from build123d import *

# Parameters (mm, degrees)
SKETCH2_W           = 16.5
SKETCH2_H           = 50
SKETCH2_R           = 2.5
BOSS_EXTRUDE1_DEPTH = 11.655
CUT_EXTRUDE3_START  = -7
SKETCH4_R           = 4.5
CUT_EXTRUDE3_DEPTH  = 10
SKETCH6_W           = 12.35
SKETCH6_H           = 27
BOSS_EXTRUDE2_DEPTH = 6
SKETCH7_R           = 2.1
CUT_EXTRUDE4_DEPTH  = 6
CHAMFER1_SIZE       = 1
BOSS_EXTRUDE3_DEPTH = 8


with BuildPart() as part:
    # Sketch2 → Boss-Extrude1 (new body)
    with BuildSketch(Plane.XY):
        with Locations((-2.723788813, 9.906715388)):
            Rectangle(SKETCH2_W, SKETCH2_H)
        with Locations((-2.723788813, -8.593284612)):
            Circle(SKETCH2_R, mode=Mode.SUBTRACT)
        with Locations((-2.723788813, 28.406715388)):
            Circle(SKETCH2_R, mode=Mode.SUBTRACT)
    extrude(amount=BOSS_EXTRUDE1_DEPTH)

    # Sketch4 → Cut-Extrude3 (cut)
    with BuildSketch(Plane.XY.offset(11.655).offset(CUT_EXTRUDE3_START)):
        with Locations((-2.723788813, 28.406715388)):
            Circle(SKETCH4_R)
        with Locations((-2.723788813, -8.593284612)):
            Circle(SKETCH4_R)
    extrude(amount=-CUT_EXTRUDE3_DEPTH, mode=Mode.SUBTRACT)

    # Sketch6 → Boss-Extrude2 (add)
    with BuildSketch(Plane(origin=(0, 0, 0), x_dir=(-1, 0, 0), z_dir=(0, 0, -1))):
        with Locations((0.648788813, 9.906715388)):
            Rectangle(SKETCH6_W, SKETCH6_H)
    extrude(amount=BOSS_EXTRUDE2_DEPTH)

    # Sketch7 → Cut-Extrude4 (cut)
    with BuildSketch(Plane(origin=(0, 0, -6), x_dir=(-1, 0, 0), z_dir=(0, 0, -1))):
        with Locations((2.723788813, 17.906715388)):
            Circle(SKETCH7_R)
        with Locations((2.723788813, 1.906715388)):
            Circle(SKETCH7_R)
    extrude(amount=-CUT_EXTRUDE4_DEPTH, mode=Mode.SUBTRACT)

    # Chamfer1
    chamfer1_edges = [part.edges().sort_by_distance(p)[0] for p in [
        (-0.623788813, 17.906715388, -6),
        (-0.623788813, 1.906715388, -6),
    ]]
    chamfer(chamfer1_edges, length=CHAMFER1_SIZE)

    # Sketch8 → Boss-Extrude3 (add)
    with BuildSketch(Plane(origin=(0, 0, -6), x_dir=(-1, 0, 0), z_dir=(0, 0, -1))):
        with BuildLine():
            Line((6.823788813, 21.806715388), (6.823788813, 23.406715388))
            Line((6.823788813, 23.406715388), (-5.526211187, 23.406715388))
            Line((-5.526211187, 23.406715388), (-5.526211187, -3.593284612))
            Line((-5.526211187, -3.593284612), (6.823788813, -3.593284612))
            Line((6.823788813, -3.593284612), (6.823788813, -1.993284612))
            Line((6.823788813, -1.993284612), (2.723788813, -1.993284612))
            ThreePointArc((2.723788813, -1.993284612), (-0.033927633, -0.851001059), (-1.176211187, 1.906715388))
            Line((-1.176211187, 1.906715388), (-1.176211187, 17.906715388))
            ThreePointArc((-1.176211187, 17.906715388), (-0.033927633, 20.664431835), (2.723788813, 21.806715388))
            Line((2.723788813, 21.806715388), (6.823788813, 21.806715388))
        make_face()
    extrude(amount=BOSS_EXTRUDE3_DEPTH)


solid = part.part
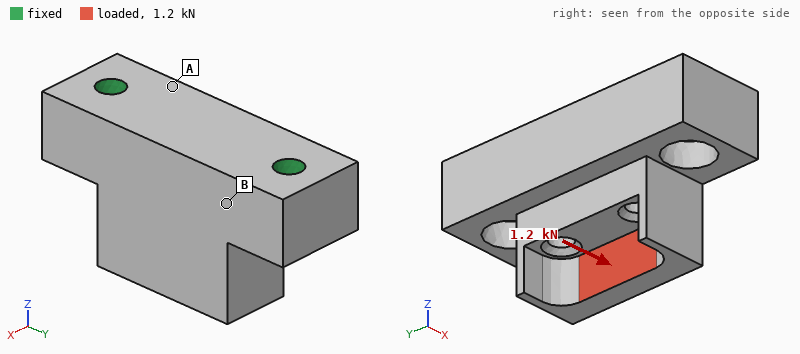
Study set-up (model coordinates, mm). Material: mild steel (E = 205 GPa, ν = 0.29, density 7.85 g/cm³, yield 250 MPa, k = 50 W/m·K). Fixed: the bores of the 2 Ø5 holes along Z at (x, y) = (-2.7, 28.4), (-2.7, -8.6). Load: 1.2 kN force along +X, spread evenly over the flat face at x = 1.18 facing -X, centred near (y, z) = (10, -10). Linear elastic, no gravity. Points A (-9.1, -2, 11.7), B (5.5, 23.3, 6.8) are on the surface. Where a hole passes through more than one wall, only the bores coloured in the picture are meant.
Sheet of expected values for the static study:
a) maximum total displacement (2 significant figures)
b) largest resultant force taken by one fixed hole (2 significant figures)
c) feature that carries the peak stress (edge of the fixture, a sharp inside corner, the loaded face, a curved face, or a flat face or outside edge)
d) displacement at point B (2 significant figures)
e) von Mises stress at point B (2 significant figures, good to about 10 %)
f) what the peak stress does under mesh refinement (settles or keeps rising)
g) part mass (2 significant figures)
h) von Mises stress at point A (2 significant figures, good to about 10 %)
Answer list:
18 µm
600 N
edge of the fixture
2.8 µm
30 MPa
keeps rising
92 g
13 MPa
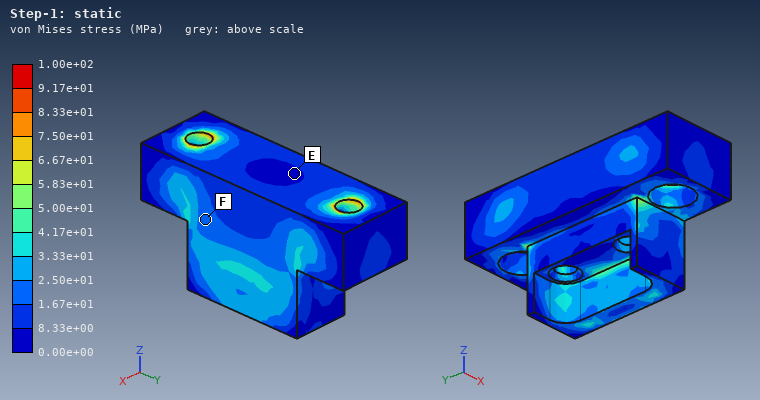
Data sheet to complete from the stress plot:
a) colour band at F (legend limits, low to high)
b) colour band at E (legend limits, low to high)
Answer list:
1.67e+01 to 2.50e+01 MPa
0.00e+00 to 8.33e+00 MPa
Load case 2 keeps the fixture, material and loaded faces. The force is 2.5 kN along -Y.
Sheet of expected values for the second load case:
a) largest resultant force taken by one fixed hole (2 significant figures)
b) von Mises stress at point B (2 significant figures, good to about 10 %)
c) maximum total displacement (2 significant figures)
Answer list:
1.8 kN
10 MPa
7.2 µm
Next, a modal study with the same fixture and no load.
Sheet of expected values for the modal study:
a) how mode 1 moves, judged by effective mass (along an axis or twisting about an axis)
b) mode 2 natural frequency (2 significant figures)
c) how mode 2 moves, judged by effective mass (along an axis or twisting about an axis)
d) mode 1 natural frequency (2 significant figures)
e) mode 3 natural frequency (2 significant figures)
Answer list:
along X
24 kHz
along Z
12 kHz
27 kHz
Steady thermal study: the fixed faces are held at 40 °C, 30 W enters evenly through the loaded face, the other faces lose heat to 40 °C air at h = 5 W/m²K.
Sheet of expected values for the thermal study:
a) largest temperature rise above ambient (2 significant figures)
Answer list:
79 K
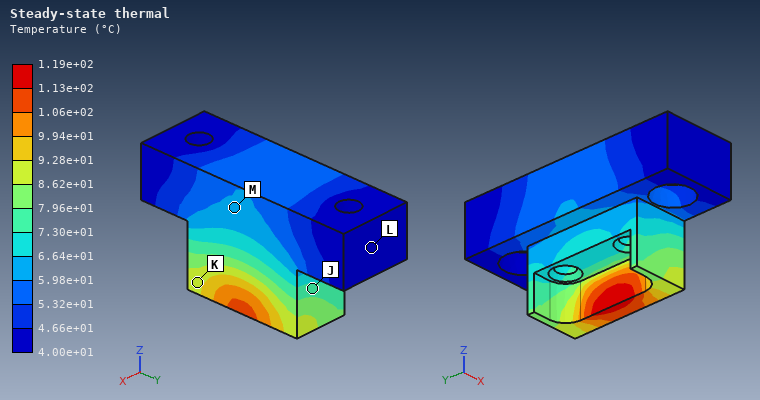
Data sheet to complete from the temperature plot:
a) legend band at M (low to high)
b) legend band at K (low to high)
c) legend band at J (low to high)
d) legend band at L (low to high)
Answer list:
5.98e+01 to 6.64e+01 °C
8.62e+01 to 9.28e+01 °C
7.30e+01 to 7.96e+01 °C
4.00e+01 to 4.66e+01 °C
